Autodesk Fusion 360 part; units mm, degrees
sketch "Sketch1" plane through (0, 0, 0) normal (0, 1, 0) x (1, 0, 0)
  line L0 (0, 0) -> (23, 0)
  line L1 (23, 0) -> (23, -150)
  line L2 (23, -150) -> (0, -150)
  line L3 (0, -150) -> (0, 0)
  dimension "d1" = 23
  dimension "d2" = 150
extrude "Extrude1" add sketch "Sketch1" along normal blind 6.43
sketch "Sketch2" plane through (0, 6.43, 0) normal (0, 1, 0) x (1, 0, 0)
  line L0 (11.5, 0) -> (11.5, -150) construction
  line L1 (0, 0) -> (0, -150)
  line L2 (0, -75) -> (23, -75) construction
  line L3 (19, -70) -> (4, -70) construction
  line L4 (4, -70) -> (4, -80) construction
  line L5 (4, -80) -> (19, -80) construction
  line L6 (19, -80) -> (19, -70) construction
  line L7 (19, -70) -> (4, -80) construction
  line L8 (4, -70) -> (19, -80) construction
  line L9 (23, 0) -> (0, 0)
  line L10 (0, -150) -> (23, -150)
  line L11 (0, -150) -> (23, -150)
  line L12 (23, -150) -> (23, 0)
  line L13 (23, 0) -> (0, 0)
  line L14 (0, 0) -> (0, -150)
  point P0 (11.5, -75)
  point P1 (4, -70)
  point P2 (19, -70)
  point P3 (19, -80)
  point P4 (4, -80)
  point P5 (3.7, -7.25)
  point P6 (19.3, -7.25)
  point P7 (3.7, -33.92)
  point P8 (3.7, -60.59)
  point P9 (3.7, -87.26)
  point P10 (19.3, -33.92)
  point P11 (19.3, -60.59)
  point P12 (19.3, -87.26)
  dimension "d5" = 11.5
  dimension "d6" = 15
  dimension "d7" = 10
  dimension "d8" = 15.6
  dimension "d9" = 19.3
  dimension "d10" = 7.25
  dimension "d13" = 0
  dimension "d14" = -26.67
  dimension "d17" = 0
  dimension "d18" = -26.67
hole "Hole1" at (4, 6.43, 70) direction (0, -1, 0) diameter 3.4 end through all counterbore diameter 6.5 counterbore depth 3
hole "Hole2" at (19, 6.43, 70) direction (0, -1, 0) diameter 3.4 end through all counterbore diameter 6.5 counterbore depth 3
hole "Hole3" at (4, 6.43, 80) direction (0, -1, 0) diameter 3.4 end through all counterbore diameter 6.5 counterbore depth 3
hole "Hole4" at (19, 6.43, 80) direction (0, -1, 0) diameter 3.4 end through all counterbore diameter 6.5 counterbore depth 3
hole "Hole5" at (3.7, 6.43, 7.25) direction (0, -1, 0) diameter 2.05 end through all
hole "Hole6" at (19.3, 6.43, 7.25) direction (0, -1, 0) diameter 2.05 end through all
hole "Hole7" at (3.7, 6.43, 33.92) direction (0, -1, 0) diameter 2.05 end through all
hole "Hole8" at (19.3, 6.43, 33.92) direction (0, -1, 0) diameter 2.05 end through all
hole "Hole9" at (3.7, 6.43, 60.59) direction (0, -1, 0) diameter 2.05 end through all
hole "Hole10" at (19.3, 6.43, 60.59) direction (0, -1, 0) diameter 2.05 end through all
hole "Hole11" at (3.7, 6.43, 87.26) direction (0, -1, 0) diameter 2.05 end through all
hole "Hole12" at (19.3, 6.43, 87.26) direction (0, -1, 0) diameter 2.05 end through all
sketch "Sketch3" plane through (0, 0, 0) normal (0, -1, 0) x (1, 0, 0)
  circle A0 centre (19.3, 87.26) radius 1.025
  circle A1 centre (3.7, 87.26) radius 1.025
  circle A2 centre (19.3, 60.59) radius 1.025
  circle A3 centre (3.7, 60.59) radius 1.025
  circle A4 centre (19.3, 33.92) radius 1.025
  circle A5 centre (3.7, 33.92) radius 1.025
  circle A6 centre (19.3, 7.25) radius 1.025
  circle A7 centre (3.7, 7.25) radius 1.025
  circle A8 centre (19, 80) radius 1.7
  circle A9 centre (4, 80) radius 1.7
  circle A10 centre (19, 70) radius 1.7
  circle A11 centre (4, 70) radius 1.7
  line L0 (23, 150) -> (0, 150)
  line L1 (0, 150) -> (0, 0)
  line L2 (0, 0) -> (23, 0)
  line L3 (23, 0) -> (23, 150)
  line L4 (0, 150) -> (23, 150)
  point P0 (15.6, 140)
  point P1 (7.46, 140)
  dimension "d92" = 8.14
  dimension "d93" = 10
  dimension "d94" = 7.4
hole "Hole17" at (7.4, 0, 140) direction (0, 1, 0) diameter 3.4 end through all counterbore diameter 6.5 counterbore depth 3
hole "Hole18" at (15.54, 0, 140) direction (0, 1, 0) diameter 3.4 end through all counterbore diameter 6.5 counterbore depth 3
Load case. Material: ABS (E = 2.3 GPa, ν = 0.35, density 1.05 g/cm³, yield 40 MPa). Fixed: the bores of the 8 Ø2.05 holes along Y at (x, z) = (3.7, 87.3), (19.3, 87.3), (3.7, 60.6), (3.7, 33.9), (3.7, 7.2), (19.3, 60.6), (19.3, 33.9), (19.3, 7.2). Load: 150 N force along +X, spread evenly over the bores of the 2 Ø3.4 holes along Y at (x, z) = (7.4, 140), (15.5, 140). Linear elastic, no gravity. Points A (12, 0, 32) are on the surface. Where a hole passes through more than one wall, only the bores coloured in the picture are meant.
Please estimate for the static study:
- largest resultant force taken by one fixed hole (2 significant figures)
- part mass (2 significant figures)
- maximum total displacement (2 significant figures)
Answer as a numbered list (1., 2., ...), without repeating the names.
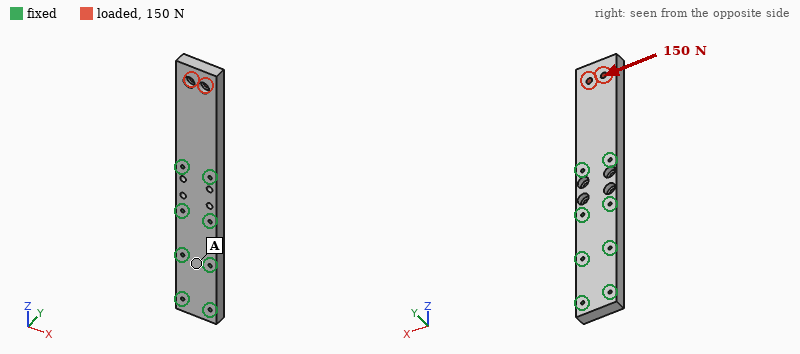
1. 460 N
2. 22 g
3. 0.78 mm
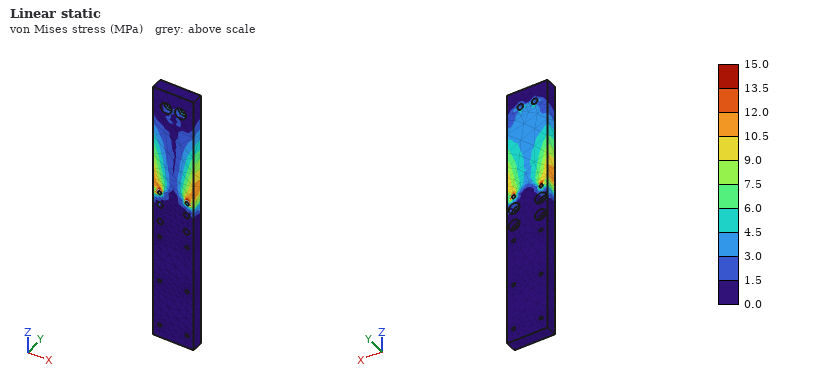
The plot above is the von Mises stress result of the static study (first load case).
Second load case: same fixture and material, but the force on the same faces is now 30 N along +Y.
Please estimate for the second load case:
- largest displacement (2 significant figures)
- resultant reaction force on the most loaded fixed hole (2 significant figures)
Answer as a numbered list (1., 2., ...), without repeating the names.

1. 1.7 mm
2. 23 N
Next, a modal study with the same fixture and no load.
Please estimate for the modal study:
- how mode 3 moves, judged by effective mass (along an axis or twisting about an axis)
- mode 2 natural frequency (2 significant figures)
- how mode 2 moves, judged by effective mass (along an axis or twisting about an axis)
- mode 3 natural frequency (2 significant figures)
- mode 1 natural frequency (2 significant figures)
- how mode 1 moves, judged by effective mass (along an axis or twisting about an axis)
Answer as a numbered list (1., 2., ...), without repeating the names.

1. twisting about Z
2. 1300 Hz
3. along X
4. 1900 Hz
5. 390 Hz
6. along Y
